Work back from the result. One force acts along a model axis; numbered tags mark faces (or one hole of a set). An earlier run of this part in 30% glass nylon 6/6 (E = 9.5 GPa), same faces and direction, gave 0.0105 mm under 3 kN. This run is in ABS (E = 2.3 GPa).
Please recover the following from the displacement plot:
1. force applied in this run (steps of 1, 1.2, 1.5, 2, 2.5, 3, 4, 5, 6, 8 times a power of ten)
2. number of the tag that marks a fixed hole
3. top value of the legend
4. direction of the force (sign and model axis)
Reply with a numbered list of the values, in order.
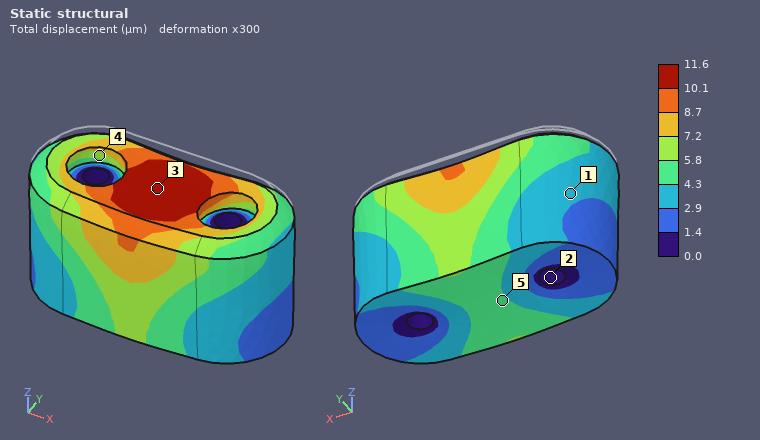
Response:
1. 800 N
2. 2
3. 11.6 µm
4. -Z
